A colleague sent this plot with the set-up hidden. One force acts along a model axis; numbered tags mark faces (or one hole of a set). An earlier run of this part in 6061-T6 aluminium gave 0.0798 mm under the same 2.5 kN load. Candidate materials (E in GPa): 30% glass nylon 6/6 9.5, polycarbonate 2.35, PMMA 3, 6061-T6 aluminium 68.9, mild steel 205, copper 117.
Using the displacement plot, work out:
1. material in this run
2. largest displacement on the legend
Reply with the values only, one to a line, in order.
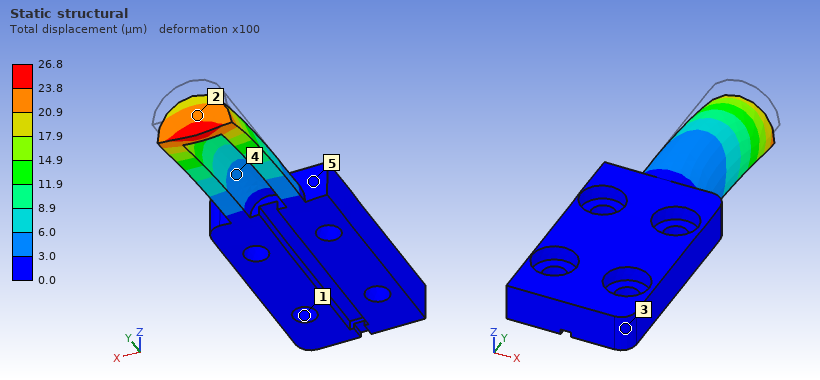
mild steel
26.8 µm
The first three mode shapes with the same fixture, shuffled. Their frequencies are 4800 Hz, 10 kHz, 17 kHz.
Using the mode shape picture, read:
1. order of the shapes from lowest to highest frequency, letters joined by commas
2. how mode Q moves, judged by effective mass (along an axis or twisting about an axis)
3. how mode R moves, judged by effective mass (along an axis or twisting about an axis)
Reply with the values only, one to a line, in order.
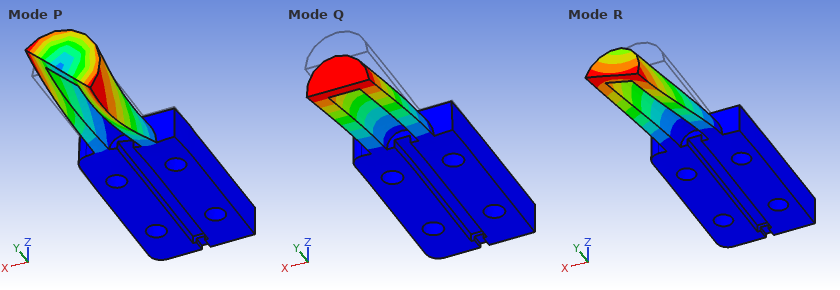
Q, R, P
along Z
along X
